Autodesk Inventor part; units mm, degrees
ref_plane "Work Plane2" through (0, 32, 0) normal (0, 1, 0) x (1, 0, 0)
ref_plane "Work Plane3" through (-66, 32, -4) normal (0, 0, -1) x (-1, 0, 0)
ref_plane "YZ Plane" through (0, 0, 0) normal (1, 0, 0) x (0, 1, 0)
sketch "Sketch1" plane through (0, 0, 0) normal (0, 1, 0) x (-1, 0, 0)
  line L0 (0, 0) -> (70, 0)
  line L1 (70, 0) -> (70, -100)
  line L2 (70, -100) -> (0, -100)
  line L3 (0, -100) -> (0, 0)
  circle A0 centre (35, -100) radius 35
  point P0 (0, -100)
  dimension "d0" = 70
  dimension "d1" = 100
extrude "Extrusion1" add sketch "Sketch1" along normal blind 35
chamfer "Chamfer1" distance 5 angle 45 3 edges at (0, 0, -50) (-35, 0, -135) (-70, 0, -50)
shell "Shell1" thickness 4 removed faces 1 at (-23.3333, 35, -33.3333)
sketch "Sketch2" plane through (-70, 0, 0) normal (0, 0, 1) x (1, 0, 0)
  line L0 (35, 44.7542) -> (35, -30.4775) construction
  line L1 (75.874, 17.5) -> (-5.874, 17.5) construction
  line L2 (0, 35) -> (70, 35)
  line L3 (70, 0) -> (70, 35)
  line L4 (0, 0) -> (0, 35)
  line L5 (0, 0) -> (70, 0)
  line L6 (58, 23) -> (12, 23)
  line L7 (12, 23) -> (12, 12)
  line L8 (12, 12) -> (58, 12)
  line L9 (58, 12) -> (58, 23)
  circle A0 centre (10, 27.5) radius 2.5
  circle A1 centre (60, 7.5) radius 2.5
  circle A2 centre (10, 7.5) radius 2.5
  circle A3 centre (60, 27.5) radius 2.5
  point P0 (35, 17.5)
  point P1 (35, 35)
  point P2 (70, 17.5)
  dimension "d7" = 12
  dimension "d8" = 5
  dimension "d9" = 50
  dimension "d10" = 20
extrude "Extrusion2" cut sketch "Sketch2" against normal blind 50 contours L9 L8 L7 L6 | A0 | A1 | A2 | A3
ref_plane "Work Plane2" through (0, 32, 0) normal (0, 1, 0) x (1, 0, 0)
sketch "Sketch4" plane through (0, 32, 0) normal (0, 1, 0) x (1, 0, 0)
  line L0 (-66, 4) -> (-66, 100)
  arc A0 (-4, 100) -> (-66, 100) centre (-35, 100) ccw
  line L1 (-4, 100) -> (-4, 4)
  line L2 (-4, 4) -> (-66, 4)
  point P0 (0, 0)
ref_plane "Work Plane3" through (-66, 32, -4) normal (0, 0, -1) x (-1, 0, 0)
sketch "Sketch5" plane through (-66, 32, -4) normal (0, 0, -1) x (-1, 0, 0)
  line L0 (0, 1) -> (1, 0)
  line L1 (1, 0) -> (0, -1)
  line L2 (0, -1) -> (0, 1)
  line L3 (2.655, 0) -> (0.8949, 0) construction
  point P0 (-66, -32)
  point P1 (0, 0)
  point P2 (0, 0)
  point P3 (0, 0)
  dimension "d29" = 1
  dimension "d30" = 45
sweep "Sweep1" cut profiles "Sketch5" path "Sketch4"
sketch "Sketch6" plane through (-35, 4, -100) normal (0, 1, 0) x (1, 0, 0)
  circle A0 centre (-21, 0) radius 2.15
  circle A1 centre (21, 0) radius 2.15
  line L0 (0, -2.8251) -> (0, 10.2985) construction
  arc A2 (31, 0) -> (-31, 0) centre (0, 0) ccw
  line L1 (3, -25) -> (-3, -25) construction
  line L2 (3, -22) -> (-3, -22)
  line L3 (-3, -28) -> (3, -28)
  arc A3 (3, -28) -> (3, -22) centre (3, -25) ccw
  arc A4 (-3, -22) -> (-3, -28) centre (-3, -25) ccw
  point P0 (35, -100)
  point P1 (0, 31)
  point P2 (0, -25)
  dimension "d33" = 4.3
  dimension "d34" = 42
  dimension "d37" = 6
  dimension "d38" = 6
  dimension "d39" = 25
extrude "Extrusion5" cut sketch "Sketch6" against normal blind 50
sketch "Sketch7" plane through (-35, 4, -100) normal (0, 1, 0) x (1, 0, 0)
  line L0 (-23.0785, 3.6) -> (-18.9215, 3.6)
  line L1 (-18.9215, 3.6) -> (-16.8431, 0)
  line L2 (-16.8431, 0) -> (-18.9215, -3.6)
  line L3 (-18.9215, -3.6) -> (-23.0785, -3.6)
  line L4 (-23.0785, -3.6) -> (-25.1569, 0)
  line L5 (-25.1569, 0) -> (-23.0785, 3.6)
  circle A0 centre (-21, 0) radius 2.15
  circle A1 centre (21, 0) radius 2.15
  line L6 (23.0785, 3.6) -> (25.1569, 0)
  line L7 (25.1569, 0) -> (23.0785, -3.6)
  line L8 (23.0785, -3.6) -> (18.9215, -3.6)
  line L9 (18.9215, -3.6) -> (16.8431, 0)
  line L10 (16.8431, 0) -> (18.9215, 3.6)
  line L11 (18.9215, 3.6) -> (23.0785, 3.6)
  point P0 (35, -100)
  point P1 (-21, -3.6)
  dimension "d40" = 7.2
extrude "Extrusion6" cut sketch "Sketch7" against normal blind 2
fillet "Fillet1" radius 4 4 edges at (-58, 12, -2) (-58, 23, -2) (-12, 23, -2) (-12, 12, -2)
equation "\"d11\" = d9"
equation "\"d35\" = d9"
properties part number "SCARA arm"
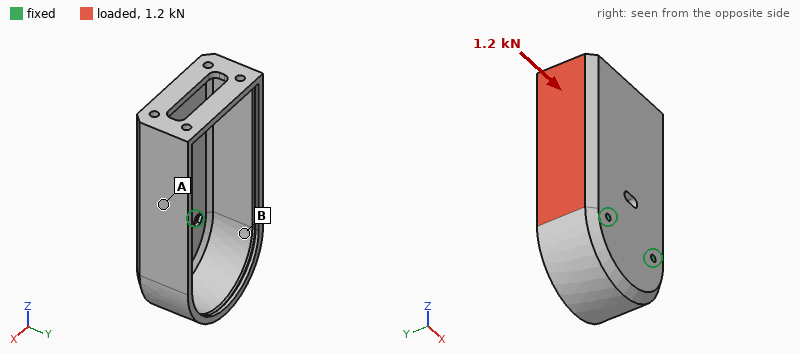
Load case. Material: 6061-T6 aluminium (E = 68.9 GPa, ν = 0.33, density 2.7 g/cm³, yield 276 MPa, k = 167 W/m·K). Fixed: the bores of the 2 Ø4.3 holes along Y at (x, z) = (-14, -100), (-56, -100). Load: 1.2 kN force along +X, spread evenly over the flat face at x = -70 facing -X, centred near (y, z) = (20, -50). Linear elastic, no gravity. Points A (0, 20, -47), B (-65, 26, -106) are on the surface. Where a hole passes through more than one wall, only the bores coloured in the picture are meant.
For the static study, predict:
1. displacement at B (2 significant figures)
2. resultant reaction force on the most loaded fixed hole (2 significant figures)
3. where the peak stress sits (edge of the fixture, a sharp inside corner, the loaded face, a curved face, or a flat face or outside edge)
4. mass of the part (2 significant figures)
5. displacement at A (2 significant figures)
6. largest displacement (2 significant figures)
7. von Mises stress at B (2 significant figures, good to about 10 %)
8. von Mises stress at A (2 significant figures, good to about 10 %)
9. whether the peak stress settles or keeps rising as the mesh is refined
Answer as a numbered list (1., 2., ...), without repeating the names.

1. 0.071 mm
2. 1.6 kN
3. edge of the fixture
4. 200 g
5. 0.10 mm
6. 0.40 mm
7. 45 MPa
8. 16 MPa
9. keeps rising
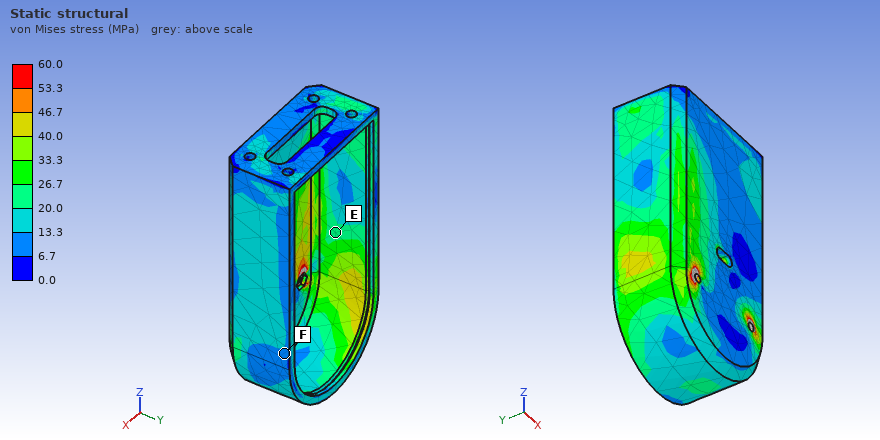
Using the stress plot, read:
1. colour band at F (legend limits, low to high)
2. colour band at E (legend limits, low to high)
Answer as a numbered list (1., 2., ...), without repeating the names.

1. 6.7 to 13.3 MPa
2. 20.0 to 26.7 MPa
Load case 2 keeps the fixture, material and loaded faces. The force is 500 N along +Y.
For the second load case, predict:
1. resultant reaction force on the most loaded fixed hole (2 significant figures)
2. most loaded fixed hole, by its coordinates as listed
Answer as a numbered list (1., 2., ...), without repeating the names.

1. 690 N
2. (-56, -100)
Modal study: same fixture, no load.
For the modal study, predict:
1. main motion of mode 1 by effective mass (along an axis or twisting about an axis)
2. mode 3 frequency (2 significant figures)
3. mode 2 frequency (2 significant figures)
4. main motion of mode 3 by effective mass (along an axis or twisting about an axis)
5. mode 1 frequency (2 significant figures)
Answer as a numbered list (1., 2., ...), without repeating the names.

1. along Y
2. 2100 Hz
3. 880 Hz
4. along X
5. 270 Hz
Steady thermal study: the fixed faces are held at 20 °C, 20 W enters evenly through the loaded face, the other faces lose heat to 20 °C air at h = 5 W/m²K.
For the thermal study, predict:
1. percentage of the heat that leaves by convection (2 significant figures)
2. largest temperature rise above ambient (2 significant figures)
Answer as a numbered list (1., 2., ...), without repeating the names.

1. 10 %
2. 22 K
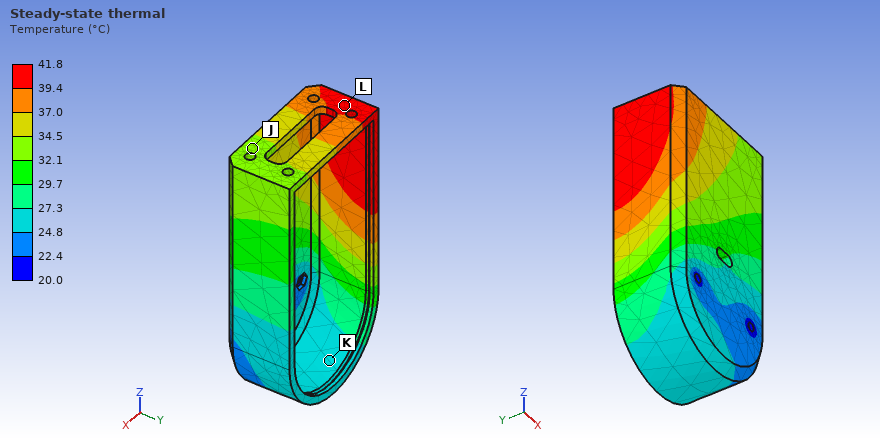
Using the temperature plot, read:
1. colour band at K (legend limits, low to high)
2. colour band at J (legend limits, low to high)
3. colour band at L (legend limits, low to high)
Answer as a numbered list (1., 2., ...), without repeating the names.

1. 24.8 to 27.3 °C
2. 32.1 to 34.5 °C
3. 39.4 to 41.8 °C
